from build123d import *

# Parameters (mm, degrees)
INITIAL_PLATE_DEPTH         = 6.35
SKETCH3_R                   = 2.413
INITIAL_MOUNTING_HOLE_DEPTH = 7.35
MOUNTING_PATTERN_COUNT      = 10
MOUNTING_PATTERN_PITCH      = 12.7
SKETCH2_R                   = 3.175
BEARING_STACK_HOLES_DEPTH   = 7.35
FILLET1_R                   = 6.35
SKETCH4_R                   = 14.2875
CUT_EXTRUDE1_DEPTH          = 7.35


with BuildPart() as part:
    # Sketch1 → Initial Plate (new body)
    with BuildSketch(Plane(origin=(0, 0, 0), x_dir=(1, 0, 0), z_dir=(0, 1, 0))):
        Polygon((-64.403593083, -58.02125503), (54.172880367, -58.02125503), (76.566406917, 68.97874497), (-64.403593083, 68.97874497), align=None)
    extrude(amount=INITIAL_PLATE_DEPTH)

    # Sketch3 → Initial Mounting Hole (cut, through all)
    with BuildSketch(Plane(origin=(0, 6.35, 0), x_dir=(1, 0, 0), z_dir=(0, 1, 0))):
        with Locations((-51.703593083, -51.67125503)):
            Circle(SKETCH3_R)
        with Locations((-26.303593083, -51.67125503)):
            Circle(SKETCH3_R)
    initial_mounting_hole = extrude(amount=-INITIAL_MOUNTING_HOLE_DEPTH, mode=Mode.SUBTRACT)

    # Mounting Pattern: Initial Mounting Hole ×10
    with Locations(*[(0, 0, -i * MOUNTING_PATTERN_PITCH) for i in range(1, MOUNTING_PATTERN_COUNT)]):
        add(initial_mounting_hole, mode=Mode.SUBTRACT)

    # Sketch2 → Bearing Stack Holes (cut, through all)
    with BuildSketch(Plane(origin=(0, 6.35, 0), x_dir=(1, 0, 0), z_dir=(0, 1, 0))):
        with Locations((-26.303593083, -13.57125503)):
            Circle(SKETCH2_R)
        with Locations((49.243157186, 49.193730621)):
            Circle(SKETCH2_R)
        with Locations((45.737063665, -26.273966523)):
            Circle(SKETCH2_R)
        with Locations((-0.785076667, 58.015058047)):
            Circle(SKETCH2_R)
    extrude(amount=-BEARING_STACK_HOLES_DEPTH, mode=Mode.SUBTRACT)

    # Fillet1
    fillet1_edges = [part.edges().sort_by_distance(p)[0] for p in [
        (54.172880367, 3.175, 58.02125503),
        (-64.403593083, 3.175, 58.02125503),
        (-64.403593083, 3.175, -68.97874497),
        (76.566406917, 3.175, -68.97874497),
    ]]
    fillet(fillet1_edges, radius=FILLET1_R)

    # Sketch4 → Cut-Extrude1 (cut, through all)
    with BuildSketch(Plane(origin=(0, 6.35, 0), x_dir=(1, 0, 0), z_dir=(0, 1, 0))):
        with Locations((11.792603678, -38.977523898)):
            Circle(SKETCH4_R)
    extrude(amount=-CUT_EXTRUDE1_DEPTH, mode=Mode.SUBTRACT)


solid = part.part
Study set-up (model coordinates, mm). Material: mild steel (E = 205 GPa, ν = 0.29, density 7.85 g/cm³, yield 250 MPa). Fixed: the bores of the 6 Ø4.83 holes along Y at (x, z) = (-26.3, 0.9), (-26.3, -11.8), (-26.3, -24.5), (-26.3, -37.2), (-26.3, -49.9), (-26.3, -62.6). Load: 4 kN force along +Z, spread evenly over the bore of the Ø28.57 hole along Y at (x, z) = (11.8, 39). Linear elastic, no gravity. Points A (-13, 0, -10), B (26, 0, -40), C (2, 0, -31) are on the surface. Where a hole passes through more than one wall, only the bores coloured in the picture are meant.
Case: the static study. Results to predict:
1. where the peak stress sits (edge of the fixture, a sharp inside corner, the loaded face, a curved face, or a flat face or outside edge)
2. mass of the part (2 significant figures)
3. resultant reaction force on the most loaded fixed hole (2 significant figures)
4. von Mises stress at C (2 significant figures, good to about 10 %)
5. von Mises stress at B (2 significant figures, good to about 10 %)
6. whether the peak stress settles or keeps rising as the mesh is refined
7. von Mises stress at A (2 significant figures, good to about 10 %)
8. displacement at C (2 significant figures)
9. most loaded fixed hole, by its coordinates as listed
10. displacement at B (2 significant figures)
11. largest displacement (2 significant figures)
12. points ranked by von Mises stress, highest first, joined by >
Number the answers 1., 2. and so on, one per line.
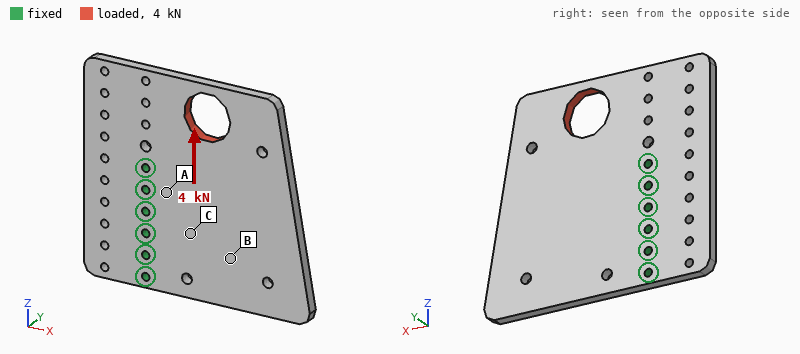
1. edge of the fixture
2. 760 g
3. 2.6 kN
4. 12 MPa
5. 5.6 MPa
6. keeps rising
7. 17 MPa
8. 3.0 µm
9. (-26.3, 0.9)
10. 5.8 µm
11. 14 µm
12. A > C > B
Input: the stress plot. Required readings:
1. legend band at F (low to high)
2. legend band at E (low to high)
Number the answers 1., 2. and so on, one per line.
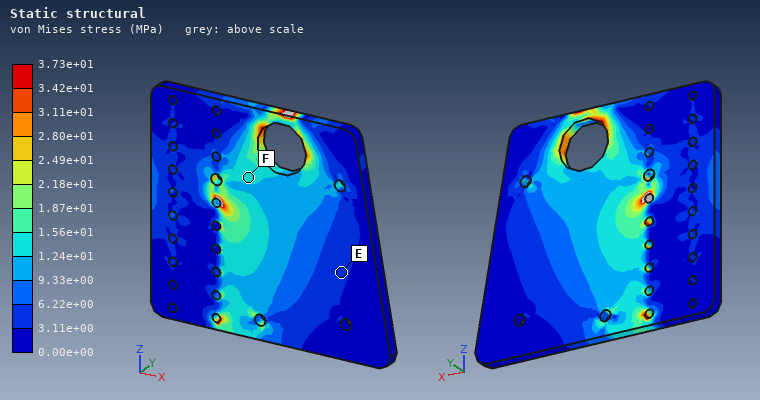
1. 1.24e+01 to 1.56e+01 MPa
2. 3.11e+00 to 6.22e+00 MPa
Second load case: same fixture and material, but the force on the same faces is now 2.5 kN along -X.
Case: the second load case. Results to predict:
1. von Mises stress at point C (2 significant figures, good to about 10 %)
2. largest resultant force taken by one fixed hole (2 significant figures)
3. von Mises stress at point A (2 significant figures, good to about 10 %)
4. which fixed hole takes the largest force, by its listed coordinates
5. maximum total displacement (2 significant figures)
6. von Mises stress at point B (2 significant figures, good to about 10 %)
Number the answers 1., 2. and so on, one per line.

1. 5.7 MPa
2. 3.2 kN
3. 10 MPa
4. (-26.3, 0.9)
5. 13 µm
6. 3.9 MPa
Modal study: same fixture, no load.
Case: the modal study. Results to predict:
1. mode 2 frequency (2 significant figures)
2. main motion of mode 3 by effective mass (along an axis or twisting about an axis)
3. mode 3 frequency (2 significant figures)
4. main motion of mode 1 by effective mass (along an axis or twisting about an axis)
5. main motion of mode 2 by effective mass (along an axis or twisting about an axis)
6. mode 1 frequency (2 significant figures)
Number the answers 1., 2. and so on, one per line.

1. 980 Hz
2. along Y
3. 1500 Hz
4. along Y
5. twisting about X
6. 560 Hz
